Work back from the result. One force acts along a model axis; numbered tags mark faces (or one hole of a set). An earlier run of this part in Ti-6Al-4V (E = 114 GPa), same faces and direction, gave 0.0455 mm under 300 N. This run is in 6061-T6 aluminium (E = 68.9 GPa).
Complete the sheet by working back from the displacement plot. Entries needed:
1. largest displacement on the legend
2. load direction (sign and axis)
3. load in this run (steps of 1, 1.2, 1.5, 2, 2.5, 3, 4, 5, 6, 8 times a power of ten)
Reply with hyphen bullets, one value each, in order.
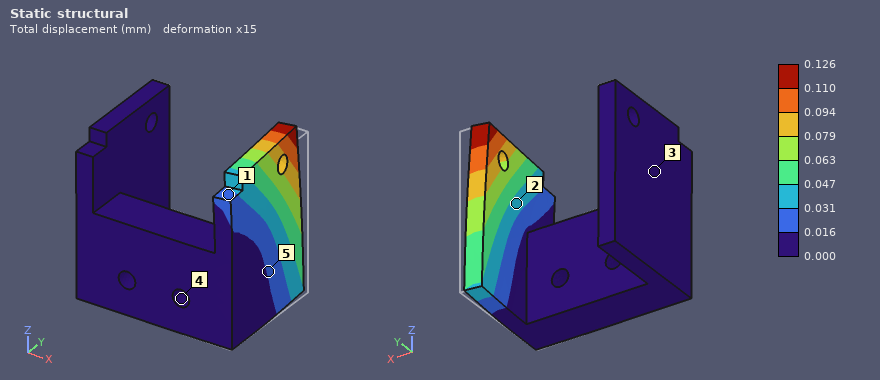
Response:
- 0.126 mm
- -X
- 500 N
